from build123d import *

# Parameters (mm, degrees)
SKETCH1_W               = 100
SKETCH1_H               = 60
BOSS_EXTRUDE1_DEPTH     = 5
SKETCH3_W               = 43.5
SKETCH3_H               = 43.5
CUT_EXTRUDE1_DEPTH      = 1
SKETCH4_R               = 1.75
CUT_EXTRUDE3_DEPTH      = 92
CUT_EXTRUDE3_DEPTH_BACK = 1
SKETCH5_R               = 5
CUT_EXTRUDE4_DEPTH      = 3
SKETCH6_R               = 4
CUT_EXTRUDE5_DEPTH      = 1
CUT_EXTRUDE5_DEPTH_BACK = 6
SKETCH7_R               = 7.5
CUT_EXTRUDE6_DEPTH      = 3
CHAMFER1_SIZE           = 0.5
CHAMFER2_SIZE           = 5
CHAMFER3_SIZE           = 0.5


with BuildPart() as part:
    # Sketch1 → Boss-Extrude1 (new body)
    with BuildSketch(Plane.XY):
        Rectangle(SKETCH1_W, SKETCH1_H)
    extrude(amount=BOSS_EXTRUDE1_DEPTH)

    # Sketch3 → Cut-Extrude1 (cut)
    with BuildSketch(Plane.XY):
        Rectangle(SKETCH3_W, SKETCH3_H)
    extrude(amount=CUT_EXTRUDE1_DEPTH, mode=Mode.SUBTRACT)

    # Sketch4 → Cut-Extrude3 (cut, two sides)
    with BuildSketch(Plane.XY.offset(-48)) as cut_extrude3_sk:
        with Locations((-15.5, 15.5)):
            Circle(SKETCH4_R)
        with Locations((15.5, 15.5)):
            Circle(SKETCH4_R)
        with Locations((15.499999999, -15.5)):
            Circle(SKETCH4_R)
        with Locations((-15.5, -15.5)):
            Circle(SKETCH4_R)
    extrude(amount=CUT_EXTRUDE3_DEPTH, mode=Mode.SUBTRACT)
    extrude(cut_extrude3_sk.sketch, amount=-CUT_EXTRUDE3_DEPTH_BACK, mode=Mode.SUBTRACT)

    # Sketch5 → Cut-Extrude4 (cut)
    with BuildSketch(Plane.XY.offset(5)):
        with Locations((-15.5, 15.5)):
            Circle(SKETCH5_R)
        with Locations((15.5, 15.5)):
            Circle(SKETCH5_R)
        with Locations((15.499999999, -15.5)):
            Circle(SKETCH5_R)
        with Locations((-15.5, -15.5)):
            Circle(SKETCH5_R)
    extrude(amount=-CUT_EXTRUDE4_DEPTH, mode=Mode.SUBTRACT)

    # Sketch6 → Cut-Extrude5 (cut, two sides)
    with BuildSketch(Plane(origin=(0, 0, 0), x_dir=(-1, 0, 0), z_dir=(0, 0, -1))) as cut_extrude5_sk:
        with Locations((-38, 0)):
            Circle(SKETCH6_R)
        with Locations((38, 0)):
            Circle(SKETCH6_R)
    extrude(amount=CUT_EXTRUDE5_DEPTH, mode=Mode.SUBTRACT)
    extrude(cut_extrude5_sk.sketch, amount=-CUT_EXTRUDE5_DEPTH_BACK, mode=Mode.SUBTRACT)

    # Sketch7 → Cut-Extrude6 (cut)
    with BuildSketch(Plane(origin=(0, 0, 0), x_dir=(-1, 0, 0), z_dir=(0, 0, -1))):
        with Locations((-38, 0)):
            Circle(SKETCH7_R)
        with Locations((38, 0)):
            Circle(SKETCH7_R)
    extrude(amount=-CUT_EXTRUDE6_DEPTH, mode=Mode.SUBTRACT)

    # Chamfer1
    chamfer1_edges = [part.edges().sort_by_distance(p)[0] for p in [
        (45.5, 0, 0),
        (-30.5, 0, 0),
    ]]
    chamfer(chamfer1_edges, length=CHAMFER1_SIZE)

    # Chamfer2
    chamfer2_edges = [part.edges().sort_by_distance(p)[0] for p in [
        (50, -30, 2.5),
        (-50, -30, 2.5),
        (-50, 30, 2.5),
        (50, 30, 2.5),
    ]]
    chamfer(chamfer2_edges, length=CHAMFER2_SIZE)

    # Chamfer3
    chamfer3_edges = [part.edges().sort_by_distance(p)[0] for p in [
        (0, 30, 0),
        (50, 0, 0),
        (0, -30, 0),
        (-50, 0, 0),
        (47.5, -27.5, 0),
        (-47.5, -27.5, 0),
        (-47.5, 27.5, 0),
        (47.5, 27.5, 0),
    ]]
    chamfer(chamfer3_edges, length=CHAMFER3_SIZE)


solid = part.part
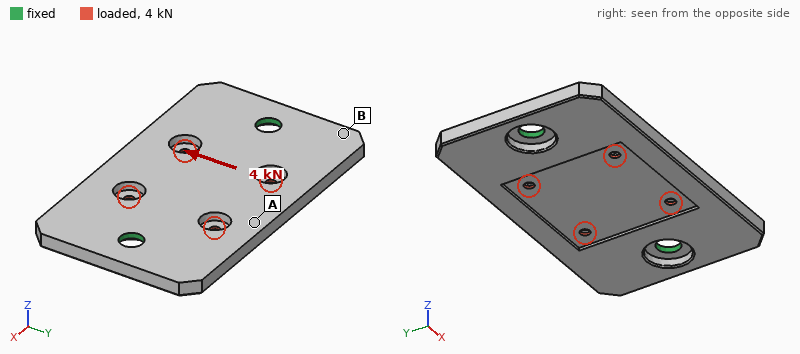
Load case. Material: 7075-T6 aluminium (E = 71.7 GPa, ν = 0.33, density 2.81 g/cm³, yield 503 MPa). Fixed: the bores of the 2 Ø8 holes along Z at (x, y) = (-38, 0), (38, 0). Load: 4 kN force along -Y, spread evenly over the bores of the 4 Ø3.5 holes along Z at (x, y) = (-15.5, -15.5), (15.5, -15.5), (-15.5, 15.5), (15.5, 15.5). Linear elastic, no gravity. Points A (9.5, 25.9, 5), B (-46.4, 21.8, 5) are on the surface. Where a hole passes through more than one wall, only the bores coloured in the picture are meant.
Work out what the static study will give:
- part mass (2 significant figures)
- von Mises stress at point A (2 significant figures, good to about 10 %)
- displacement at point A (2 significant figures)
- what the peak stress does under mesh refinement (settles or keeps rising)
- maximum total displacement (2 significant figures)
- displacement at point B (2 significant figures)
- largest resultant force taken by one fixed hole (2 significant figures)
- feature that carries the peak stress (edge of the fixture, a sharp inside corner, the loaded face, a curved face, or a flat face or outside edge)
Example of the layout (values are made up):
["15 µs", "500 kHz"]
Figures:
["72 g", "23 MPa", "0.10 mm", "keeps rising", "0.12 mm", "0.062 mm", "2.0 kN", "edge of the fixture"]
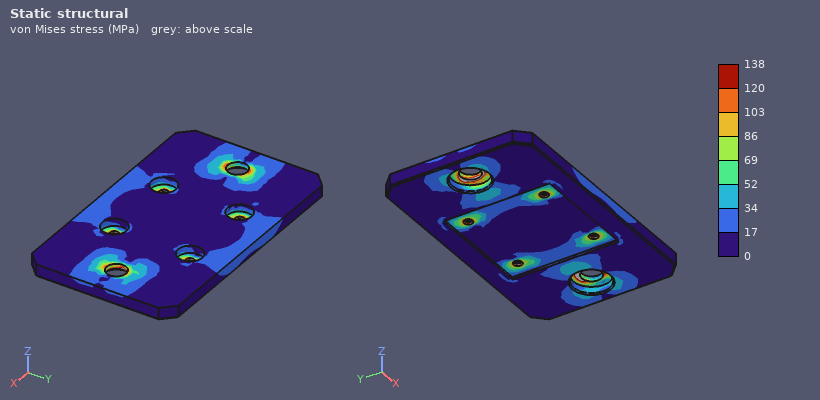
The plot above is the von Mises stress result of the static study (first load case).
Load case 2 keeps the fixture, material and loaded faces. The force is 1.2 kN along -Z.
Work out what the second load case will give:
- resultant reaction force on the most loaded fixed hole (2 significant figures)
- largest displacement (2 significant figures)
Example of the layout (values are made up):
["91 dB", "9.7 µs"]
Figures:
["1.2 kN", "0.15 mm"]
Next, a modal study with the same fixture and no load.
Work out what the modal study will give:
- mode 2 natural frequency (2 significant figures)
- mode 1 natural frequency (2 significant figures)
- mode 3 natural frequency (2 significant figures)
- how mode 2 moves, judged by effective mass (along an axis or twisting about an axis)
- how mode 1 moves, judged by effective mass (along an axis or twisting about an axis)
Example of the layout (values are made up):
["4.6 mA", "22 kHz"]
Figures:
["2600 Hz", "1800 Hz", "3500 Hz", "along Z", "twisting about X"]
